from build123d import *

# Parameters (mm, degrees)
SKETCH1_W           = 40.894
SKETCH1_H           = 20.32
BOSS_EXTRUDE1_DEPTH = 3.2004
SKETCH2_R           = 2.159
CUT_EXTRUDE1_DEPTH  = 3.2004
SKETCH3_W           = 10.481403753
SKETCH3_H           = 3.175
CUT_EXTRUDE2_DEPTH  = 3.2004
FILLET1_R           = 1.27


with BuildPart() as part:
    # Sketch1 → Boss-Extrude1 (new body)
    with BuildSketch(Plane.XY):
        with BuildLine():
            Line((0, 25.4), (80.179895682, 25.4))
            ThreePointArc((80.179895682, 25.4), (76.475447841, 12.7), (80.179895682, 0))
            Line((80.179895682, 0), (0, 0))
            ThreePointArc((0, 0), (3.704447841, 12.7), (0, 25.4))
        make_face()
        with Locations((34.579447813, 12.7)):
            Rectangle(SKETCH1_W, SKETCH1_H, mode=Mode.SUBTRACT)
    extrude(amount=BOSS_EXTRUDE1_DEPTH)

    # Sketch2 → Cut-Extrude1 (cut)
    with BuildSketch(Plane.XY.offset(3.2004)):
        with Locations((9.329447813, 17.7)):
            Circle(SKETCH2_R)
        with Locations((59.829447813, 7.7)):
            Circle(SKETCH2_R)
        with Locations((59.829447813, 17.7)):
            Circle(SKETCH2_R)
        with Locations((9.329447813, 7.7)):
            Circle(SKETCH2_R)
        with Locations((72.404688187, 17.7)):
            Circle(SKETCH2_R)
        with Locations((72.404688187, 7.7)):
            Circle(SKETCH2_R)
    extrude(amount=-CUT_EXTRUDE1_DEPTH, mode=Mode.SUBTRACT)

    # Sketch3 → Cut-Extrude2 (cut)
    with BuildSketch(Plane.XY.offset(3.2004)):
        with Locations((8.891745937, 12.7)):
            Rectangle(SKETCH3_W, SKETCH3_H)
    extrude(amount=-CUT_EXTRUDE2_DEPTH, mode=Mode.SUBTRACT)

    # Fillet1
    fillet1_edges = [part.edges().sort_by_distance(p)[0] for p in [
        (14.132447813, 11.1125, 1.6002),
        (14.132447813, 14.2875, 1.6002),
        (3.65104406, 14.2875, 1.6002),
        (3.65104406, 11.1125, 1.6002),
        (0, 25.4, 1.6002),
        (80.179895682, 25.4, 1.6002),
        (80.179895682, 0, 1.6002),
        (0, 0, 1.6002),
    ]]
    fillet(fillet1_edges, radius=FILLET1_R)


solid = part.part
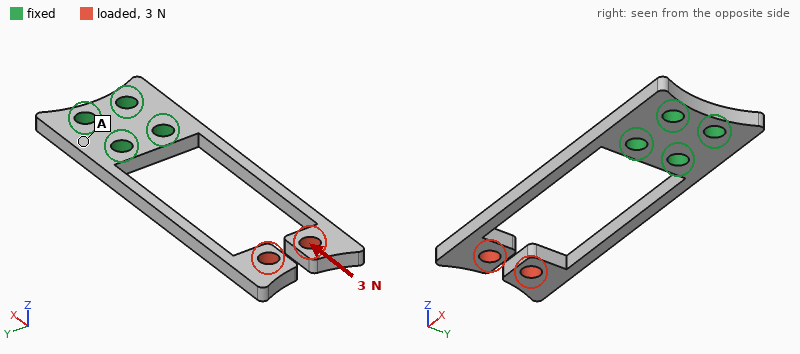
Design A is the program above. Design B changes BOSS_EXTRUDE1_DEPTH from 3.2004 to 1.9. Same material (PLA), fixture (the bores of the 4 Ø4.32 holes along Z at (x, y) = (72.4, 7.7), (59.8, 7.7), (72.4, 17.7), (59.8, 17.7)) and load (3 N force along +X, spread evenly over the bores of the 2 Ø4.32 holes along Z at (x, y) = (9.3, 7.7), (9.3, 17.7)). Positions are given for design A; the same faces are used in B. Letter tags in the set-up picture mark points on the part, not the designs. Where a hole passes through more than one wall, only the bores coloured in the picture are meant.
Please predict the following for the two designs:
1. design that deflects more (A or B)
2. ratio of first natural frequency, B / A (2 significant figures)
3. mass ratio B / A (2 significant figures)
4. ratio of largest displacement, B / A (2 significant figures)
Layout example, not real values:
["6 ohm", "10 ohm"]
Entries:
["B", "0.72", "0.59", "1.7"]
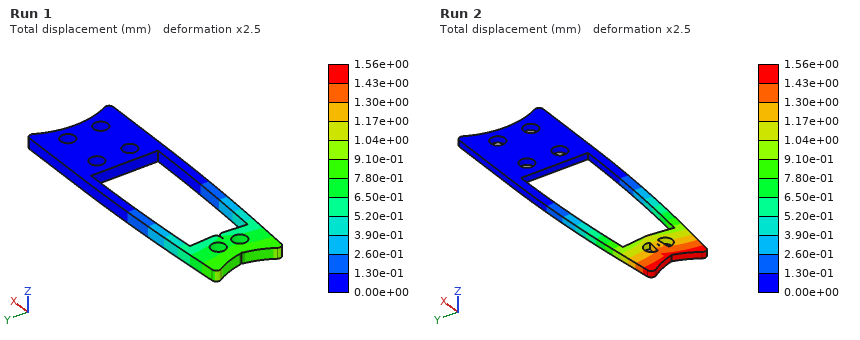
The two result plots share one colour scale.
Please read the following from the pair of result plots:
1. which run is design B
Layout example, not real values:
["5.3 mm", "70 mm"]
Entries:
["Run 2"]
